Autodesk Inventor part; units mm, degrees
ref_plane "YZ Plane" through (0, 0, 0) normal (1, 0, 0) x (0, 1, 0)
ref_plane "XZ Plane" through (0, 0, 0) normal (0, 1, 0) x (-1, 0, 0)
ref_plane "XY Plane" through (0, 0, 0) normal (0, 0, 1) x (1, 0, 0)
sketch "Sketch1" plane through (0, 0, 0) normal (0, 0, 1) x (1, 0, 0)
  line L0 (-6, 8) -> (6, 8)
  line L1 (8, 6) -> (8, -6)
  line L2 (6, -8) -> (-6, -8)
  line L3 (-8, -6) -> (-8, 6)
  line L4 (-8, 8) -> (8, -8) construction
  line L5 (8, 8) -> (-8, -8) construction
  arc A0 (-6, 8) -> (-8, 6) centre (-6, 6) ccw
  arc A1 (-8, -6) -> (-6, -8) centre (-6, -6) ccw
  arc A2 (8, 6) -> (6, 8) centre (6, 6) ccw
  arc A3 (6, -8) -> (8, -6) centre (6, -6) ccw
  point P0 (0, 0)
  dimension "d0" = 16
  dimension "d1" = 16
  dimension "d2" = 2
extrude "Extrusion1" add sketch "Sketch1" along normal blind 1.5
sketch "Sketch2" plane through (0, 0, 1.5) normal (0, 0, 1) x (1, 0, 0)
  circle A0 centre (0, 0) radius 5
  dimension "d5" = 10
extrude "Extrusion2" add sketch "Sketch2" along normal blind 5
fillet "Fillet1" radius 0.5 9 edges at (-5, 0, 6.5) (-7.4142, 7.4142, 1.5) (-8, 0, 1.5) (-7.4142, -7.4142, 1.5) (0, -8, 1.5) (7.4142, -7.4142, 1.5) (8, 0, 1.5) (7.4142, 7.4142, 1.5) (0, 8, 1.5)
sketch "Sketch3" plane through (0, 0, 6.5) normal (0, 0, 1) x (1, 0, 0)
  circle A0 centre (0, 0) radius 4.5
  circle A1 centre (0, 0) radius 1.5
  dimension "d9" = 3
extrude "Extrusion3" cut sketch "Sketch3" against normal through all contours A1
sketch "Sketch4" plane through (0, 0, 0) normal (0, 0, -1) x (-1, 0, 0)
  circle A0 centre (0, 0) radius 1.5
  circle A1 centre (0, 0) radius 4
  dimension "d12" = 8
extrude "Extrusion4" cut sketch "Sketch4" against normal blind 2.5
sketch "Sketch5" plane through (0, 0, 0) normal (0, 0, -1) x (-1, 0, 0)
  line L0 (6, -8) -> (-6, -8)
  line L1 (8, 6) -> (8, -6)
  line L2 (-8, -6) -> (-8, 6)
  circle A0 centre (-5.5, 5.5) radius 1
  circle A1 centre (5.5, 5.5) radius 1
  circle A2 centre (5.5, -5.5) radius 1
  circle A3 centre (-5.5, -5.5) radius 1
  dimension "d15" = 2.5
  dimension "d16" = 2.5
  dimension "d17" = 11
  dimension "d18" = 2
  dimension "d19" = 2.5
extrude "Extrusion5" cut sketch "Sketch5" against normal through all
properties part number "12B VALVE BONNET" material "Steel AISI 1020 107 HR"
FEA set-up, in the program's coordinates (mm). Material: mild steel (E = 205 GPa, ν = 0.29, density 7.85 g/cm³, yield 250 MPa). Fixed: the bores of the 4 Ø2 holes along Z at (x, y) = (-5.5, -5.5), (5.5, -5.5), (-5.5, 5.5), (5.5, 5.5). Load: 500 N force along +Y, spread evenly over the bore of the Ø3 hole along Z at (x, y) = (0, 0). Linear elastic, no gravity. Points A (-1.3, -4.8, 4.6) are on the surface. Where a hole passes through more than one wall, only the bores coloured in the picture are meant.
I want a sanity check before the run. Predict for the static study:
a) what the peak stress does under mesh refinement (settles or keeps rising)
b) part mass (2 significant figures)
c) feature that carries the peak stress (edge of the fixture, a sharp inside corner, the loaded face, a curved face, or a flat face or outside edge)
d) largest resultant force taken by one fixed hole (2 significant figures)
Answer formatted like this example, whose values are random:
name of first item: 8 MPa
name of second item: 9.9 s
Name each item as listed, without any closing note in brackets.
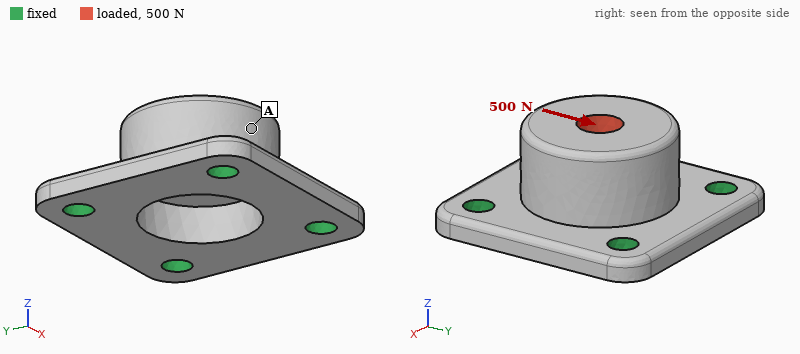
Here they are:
what the peak stress does under mesh refinement: keeps rising
part mass: 4.7 g
feature that carries the peak stress: edge of the fixture
largest resultant force taken by one fixed hole: 160 N
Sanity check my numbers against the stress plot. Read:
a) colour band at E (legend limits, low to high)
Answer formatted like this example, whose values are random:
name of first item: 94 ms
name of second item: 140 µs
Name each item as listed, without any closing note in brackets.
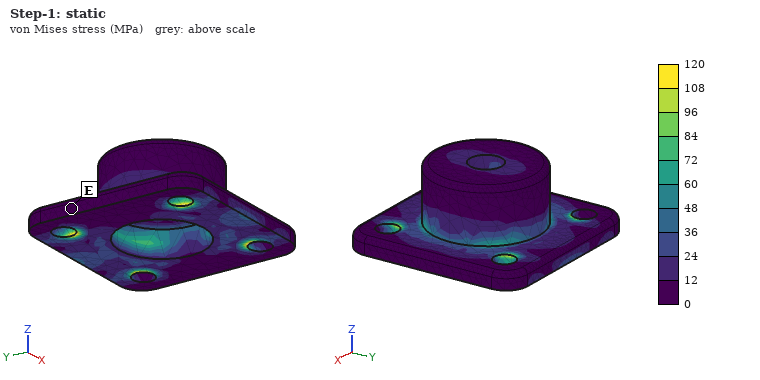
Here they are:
colour band at E: 0 to 12 MPa
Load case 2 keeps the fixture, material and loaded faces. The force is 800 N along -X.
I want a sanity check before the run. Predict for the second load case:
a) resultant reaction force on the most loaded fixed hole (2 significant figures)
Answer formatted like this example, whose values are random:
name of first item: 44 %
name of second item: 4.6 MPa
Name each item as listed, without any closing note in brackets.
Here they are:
resultant reaction force on the most loaded fixed hole: 260 N
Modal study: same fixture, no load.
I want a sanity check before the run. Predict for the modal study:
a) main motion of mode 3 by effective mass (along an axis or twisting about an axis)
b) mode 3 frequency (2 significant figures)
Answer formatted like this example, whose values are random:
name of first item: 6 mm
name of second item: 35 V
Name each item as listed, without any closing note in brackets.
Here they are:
main motion of mode 3 by effective mass: along Z
mode 3 frequency: 46 kHz
